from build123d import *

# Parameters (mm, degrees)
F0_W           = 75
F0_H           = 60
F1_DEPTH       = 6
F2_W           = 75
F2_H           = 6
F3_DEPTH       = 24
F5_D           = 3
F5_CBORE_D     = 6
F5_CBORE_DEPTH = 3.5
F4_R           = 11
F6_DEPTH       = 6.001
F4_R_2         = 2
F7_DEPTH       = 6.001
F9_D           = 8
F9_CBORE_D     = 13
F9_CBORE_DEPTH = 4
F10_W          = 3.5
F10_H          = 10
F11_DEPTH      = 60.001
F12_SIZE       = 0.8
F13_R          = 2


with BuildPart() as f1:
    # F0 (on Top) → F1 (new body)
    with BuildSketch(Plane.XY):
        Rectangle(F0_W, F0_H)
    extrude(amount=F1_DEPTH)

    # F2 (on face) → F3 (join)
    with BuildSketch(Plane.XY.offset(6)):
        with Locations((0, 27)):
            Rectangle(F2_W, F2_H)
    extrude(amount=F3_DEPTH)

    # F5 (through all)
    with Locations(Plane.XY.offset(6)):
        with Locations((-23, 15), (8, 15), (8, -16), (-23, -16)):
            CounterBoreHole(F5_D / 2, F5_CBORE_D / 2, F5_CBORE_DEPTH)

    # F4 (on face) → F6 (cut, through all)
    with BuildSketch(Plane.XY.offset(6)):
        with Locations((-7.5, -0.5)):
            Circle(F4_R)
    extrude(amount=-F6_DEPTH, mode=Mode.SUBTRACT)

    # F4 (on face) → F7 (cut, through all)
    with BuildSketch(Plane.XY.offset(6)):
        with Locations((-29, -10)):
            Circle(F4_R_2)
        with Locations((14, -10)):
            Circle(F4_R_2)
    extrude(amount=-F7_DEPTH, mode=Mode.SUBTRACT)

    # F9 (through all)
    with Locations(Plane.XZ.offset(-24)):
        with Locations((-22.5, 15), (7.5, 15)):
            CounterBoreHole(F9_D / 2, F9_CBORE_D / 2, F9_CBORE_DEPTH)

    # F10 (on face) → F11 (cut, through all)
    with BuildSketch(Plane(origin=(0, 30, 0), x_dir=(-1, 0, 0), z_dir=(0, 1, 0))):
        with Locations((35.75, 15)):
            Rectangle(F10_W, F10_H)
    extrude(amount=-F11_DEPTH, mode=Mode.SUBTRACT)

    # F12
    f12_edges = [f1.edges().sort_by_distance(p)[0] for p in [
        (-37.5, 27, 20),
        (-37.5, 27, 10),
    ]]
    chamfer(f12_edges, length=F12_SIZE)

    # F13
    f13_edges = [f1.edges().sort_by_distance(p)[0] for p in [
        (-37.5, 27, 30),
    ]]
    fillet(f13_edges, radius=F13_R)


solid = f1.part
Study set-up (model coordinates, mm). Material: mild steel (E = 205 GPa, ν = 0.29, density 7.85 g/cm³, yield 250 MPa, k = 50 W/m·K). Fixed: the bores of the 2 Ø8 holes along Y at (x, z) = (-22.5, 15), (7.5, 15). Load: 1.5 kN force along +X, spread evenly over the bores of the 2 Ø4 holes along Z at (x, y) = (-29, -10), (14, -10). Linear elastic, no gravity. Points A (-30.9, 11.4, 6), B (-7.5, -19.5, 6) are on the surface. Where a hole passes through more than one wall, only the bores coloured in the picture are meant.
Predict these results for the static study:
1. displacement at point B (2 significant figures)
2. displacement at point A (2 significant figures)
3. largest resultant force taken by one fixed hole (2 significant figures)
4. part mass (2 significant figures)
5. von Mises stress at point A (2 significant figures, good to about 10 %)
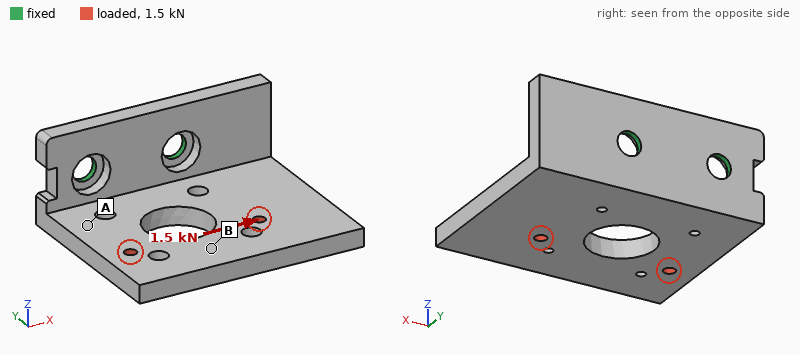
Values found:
43 µm
25 µm
2.1 kN
260 g
30 MPa
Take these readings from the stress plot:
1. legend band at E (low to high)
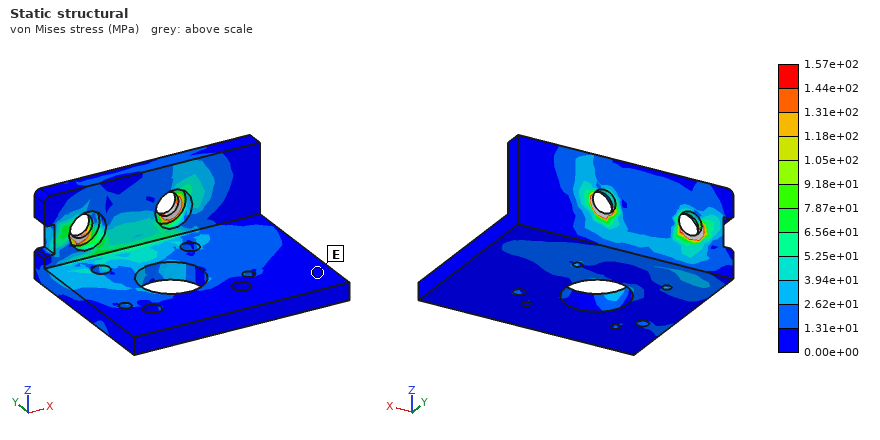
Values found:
0.00e+00 to 1.31e+01 MPa
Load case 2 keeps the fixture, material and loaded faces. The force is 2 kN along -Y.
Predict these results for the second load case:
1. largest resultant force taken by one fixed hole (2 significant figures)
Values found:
1.0 kN
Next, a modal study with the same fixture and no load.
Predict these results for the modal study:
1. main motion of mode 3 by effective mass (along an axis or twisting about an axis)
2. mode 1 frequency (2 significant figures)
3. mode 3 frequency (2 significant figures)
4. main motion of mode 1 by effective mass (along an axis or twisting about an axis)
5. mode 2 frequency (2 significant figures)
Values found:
along X
850 Hz
2800 Hz
along Z
2000 Hz
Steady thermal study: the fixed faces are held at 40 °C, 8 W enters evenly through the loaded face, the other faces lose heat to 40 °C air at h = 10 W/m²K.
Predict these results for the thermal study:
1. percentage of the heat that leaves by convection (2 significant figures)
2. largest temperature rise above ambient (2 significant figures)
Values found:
21 %
25 K
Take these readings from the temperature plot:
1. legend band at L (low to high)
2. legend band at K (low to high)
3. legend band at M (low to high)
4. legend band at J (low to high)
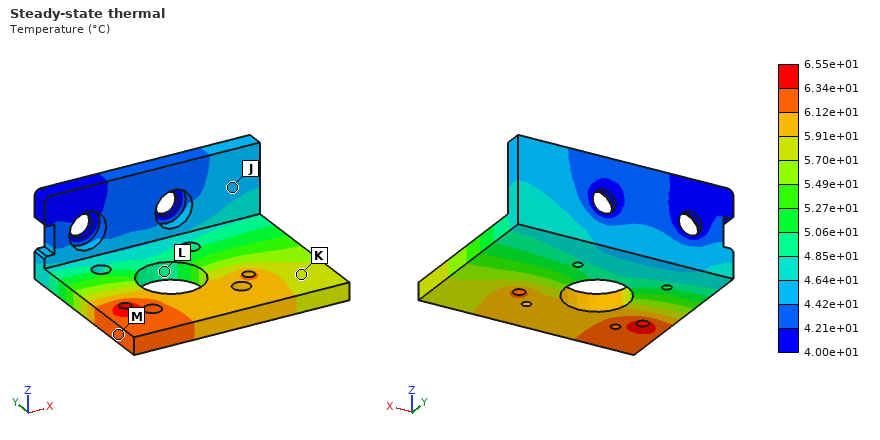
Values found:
4.85e+01 to 5.06e+01 °C
5.70e+01 to 5.91e+01 °C
6.12e+01 to 6.34e+01 °C
4.42e+01 to 4.64e+01 °C
